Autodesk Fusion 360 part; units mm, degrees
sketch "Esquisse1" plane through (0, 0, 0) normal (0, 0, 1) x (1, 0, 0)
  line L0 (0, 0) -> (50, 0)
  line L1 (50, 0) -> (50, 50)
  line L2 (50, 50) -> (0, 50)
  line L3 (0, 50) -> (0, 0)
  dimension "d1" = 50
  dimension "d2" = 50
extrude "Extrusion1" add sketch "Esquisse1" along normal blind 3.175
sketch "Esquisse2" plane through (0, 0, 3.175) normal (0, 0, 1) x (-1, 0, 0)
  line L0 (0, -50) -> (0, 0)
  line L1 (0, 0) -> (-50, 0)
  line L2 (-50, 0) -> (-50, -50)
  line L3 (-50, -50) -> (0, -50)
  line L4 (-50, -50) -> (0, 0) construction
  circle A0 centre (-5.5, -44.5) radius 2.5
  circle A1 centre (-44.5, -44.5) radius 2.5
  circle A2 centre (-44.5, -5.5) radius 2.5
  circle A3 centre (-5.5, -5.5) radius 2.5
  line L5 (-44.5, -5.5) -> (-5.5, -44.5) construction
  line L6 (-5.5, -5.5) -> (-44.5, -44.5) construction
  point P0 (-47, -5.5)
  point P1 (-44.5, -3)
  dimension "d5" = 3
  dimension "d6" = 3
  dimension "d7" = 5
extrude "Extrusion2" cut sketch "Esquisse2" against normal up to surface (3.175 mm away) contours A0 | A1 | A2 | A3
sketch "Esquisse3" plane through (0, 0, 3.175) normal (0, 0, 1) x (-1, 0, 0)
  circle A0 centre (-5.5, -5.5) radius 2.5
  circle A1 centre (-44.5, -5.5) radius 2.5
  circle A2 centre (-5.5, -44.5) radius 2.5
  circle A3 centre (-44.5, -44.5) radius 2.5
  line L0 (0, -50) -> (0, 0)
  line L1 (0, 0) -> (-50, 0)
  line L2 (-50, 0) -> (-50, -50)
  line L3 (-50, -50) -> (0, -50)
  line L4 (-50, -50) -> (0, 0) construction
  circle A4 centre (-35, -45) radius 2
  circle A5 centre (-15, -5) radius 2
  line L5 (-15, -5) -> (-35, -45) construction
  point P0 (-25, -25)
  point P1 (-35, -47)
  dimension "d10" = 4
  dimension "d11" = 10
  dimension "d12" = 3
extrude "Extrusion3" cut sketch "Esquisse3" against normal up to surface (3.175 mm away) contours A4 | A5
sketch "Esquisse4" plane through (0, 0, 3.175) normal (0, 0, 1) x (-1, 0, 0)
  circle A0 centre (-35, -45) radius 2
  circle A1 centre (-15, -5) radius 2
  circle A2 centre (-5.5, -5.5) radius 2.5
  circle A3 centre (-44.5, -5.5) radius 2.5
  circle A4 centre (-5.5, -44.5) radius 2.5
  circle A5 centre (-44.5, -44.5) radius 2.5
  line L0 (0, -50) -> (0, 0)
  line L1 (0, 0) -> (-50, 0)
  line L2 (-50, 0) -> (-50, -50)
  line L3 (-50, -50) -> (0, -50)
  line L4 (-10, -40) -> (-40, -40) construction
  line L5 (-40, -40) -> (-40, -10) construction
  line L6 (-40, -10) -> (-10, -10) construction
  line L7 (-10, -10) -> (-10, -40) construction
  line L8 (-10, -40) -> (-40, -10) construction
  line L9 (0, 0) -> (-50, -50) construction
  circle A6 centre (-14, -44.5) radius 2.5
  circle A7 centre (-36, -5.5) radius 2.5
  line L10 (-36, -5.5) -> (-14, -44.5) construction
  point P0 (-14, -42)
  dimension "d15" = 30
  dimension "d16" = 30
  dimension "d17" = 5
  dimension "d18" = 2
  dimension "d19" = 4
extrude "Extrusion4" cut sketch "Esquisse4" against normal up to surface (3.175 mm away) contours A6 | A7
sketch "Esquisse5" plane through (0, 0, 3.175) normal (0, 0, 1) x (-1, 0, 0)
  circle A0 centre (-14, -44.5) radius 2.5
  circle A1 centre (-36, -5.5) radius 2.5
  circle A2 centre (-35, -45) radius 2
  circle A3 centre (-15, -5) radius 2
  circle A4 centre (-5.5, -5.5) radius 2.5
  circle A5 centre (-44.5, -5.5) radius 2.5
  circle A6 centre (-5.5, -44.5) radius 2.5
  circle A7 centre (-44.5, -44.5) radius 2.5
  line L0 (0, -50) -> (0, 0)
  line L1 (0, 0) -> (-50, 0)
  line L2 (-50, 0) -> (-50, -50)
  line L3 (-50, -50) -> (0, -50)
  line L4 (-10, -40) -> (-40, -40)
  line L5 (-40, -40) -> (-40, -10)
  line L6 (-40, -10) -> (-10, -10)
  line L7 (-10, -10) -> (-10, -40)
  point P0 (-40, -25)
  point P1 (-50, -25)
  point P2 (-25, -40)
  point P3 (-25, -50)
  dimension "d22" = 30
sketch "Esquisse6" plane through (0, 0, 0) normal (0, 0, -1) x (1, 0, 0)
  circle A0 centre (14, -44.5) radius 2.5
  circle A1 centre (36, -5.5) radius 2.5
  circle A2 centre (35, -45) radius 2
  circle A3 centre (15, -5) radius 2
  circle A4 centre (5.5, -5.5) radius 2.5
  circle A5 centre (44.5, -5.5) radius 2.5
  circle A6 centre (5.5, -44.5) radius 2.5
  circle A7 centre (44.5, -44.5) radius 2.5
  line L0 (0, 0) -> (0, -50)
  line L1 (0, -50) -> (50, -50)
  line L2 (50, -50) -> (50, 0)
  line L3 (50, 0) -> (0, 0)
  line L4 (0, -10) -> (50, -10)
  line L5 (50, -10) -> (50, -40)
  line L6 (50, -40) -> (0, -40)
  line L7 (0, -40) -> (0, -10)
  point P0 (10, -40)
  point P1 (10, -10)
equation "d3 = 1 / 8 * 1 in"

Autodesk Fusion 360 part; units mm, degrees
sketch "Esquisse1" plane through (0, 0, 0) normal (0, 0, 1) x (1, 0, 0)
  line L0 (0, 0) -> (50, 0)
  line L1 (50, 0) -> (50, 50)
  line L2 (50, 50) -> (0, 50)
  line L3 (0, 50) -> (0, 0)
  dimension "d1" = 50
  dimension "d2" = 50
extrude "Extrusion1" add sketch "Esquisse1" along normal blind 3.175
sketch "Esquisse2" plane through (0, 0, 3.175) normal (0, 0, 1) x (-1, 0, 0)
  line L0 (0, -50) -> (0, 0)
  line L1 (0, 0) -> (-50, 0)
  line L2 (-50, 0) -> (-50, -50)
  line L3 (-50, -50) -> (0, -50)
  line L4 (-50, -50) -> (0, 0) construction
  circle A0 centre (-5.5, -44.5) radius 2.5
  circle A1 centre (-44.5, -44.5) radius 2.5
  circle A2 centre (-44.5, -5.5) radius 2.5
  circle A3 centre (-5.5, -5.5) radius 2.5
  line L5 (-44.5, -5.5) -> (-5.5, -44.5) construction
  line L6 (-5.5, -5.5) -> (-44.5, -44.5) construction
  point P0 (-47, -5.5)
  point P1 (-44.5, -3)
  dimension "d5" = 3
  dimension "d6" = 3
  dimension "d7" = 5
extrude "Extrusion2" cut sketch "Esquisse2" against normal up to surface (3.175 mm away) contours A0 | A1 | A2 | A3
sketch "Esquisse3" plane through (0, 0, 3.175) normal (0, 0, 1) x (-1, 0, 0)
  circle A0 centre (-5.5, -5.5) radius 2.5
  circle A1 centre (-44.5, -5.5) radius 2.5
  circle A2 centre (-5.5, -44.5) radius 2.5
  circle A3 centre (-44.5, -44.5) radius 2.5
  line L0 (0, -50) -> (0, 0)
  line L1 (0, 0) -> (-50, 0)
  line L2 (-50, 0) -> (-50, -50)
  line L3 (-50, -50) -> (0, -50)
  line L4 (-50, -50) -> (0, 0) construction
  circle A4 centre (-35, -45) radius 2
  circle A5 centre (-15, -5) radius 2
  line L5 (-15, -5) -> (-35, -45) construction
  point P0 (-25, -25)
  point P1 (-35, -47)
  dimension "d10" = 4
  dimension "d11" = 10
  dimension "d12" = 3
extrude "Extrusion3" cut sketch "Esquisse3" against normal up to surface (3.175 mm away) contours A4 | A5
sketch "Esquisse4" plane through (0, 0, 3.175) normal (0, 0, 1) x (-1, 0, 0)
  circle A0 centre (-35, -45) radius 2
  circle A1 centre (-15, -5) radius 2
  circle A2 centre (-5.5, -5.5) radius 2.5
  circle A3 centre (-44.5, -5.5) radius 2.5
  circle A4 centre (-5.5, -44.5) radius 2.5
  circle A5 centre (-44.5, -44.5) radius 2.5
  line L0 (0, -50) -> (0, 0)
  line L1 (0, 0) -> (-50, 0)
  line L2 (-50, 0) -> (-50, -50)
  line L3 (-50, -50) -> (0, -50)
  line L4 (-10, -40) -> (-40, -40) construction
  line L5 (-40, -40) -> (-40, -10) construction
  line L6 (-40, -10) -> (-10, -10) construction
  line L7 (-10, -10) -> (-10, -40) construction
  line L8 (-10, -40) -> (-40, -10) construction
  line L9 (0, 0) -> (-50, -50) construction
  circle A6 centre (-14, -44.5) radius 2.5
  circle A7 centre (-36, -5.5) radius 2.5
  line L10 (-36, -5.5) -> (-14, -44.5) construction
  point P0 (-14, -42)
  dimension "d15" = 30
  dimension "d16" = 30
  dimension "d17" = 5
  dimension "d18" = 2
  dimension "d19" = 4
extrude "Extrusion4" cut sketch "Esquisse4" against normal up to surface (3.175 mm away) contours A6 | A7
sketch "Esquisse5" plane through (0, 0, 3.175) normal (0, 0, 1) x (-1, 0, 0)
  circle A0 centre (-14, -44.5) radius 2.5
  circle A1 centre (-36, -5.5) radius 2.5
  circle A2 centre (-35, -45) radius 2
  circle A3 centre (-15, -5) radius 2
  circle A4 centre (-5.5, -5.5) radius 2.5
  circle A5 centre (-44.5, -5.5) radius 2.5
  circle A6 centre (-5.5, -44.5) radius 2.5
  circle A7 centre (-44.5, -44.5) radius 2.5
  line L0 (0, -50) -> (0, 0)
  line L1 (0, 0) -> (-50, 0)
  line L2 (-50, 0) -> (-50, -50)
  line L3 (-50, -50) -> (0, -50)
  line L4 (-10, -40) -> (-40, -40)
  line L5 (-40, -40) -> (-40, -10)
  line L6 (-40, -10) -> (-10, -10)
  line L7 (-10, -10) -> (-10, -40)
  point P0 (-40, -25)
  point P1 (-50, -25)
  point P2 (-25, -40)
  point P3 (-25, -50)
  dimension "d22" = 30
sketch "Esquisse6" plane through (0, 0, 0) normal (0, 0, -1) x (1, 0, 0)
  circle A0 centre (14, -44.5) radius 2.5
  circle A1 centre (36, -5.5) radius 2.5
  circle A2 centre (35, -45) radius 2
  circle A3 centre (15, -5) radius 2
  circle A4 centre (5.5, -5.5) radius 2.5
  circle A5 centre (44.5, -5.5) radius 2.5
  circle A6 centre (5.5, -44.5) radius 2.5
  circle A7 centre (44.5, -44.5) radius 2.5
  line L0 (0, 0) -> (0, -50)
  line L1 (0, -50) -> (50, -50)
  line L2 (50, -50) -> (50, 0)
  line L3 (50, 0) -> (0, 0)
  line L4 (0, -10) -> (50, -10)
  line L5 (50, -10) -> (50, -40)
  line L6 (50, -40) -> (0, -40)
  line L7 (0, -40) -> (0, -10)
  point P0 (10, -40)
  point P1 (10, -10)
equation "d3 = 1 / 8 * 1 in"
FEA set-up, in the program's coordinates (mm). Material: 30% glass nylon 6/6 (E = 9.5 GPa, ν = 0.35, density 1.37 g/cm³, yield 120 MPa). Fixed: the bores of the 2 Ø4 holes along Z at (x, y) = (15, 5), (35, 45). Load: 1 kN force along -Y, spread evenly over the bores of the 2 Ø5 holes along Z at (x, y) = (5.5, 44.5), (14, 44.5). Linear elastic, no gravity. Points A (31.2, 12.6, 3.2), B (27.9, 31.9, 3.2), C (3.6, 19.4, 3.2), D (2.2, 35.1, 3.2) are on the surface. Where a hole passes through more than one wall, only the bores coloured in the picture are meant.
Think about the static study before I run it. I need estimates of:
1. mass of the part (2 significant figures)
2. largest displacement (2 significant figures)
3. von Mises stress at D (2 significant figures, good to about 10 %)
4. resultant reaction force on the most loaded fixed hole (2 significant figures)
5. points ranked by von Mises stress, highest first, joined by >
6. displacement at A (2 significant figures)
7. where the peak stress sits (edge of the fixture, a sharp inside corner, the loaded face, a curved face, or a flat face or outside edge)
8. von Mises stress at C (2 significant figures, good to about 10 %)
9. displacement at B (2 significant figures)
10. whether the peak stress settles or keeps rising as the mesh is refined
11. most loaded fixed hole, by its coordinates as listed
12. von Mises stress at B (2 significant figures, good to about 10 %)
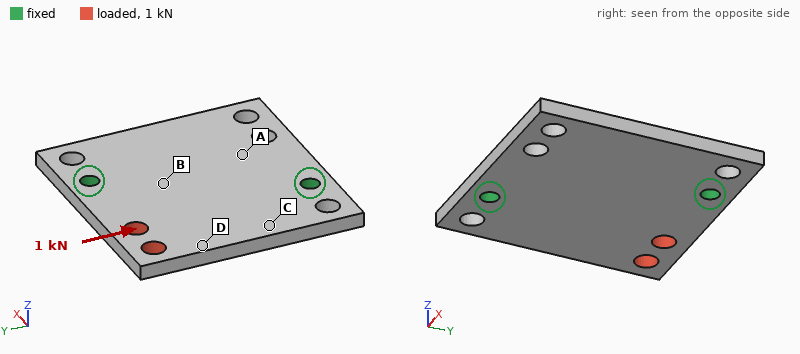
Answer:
10 g
84 µm
15 MPa
730 N
D > C > B > A
14 µm
edge of the fixture
11 MPa
15 µm
keeps rising
(15, 5)
5.5 MPa
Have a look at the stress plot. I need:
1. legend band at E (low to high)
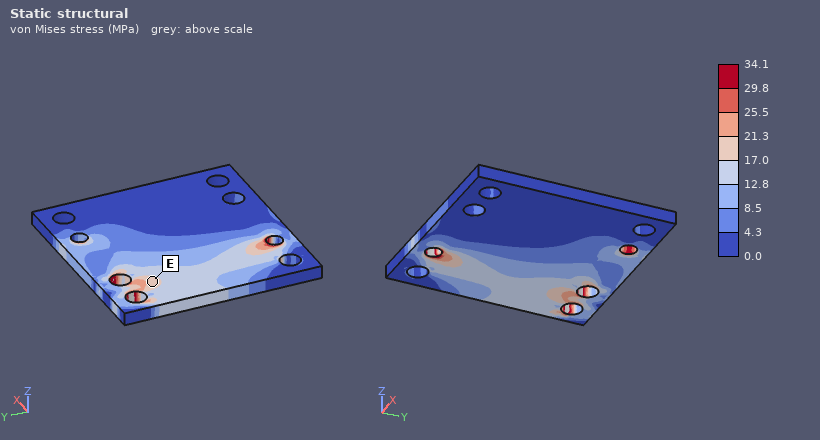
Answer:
17.0 to 21.3 MPa
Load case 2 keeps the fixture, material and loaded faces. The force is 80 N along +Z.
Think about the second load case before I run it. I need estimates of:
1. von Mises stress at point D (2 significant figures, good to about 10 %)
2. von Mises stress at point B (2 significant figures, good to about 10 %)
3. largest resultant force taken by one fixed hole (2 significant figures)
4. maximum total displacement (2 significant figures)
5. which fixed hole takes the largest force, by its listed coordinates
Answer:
10 MPa
11 MPa
63 N
0.80 mm
(35, 45)
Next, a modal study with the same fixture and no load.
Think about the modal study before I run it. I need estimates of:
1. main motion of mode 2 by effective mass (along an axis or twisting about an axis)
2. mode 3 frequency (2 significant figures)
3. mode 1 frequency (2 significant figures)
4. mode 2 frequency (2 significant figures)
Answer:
along Z
4300 Hz
1400 Hz
1900 Hz
